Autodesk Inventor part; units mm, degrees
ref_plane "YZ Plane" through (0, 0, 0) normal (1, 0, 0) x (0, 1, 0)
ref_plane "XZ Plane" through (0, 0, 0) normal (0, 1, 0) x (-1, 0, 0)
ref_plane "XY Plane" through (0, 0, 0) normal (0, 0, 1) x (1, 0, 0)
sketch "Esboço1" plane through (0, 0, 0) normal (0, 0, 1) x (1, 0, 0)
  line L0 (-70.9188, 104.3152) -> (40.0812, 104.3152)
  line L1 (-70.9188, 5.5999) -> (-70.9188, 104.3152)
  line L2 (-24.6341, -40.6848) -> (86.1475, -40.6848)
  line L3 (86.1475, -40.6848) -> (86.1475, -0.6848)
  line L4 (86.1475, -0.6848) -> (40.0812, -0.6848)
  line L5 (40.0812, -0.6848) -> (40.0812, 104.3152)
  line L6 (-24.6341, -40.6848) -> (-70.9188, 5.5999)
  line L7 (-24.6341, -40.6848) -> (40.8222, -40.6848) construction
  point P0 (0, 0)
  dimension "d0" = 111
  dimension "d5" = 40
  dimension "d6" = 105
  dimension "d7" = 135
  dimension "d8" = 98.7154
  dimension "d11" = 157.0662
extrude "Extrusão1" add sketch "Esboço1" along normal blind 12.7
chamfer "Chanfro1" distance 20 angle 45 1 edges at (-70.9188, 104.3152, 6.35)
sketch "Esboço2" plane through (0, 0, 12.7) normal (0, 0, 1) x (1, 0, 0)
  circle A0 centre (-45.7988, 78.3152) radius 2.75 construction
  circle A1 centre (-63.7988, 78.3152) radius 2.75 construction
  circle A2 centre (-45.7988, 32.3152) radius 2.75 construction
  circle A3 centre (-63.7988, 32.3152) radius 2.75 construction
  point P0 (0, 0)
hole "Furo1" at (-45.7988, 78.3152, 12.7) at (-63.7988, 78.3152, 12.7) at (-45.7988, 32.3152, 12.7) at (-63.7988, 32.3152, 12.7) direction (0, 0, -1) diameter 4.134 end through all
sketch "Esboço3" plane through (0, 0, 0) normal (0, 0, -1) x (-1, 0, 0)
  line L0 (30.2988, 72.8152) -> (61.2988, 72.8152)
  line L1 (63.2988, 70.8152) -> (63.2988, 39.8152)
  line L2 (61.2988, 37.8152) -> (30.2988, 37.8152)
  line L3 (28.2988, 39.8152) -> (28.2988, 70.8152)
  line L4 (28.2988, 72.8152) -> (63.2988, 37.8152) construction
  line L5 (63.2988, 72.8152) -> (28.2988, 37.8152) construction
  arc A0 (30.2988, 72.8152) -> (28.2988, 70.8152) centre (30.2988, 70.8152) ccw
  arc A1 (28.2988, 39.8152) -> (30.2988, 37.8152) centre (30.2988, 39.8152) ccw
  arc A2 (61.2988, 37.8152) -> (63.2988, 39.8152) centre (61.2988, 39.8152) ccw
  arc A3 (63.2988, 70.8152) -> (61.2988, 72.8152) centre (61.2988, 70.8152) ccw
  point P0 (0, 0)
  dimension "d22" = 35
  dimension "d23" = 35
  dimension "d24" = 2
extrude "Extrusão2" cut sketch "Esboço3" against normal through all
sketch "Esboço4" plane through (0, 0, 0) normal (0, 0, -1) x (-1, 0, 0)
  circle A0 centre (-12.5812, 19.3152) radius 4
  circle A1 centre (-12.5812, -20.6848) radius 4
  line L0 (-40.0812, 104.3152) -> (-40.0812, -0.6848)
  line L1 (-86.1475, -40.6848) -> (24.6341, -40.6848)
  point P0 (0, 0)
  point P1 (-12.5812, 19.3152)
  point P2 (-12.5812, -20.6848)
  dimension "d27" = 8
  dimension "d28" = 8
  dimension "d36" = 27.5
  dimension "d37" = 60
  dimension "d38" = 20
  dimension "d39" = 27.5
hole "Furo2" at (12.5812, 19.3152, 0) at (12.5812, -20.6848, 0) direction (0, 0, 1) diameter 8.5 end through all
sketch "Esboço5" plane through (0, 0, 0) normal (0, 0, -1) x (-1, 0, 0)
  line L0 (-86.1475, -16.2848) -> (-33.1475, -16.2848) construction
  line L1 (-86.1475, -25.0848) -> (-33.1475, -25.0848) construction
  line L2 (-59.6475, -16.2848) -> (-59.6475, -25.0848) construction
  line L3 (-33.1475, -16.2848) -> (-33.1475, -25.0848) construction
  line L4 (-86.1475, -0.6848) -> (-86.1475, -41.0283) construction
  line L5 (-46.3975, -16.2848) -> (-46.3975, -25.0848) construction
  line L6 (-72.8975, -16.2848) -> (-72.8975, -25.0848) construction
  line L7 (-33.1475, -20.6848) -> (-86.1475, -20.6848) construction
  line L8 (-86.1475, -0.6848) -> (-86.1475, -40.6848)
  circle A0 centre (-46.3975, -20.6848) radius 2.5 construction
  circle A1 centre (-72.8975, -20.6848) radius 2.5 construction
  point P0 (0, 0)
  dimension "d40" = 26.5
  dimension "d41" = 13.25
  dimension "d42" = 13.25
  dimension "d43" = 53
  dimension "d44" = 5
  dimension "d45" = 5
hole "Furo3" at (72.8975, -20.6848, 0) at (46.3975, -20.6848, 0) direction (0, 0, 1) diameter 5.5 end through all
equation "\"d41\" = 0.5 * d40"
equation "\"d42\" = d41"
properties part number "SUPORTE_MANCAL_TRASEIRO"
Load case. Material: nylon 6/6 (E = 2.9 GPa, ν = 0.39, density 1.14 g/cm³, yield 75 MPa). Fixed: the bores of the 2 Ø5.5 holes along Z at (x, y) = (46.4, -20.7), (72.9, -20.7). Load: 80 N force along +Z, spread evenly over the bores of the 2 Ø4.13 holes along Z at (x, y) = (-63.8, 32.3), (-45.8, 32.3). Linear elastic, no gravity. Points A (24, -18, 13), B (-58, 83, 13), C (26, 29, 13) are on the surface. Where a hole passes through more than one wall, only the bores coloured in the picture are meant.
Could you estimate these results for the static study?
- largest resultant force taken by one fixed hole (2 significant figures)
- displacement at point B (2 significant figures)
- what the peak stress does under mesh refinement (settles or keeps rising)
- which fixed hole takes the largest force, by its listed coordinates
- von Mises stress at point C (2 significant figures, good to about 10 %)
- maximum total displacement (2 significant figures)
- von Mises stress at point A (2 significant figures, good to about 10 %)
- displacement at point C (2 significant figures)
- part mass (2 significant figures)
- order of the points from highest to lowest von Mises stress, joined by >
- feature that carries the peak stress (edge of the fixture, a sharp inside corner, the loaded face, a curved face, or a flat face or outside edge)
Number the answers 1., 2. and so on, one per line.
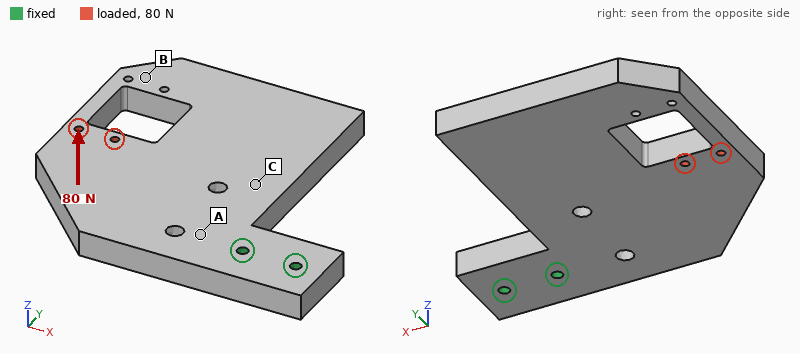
1. 210 N
2. 2.1 mm
3. keeps rising
4. (46.4, -20.7)
5. 1.9 MPa
6. 2.3 mm
7. 5.3 MPa
8. 0.37 mm
9. 220 g
10. A > C > B
11. edge of the fixture
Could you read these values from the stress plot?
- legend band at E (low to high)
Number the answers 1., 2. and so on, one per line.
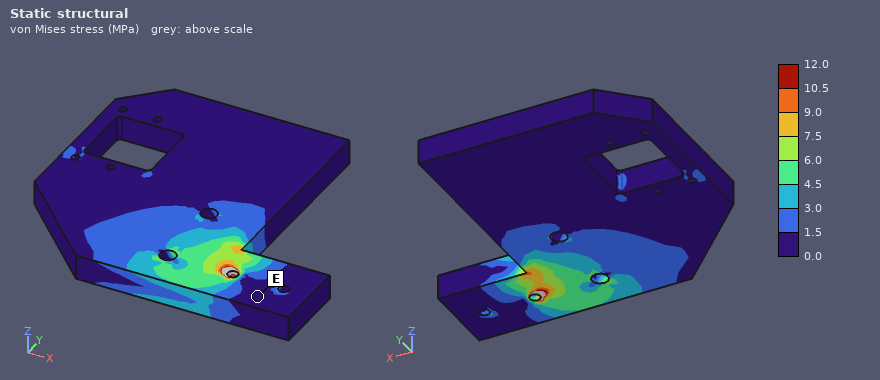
1. 0.0 to 1.5 MPa
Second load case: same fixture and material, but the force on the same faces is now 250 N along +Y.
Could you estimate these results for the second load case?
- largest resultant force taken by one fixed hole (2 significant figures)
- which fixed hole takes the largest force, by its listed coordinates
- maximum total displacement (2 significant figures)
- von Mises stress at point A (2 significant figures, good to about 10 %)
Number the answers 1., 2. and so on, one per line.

1. 1.0 kN
2. (46.4, -20.7)
3. 1.0 mm
4. 2.5 MPa
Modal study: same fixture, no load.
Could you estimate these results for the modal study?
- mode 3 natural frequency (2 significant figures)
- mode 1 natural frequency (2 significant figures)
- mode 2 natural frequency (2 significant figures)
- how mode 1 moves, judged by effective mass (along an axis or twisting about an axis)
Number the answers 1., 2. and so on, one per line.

1. 250 Hz
2. 110 Hz
3. 240 Hz
4. along Z
